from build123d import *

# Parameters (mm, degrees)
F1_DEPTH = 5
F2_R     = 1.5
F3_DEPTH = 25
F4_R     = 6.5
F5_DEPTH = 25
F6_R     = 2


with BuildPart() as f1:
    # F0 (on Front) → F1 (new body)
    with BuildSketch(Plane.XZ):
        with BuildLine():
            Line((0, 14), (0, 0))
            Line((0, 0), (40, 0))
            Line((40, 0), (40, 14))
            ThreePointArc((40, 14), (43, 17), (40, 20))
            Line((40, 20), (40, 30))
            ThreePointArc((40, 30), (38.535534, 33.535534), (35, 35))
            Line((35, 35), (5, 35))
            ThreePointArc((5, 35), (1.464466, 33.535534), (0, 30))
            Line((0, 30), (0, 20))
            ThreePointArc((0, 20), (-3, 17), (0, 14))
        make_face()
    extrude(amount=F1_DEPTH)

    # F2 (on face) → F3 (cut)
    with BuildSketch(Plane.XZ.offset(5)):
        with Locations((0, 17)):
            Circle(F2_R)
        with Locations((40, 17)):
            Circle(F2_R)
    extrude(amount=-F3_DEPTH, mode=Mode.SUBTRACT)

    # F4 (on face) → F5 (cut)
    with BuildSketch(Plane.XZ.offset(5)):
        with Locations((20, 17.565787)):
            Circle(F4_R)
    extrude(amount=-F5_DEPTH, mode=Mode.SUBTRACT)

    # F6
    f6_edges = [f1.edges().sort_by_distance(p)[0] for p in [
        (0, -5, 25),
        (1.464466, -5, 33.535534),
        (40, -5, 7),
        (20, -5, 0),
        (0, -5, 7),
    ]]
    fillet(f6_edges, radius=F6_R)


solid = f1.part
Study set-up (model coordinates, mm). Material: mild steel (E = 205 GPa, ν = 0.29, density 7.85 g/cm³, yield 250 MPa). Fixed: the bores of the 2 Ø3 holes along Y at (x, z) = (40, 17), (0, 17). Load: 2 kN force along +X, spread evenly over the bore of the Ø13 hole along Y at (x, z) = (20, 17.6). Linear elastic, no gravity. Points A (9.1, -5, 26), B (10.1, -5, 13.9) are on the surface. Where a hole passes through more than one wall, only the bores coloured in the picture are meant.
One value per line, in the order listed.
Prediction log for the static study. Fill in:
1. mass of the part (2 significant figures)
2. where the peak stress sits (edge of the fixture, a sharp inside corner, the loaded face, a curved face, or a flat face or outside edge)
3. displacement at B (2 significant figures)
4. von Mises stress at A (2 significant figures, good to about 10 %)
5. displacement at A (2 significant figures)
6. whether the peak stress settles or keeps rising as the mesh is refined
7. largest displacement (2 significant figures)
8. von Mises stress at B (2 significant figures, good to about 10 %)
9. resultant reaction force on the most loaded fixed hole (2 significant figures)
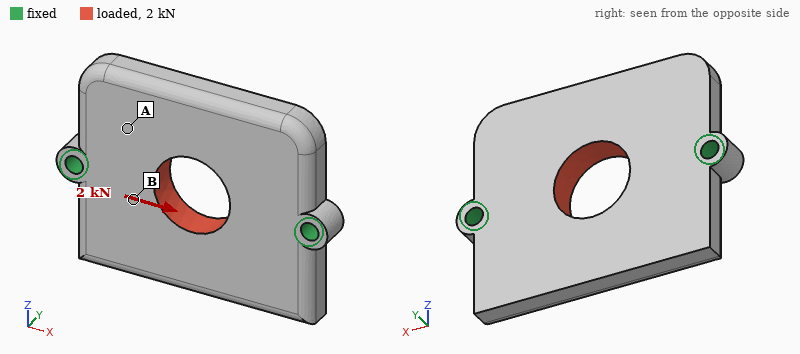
49 g
edge of the fixture
0.96 µm
5.5 MPa
1.2 µm
keeps rising
1.6 µm
14 MPa
1.0 kN
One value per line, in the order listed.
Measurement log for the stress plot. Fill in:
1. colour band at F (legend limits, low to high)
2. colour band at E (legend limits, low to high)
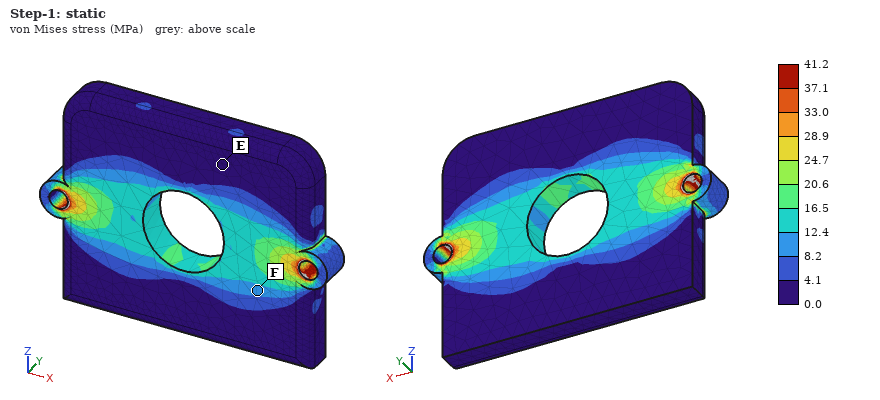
8.2 to 12.4 MPa
0.0 to 4.1 MPa
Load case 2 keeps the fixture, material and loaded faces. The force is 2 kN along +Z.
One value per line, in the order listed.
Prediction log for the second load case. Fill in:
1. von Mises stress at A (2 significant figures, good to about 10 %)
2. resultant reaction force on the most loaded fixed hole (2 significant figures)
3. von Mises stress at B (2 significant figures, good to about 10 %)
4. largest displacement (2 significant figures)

13 MPa
1.0 kN
12 MPa
2.6 µm
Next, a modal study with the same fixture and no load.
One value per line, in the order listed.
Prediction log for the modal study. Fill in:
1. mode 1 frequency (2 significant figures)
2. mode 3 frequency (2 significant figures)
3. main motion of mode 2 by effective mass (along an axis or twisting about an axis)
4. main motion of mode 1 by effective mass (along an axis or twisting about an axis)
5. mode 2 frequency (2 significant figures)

6500 Hz
15 kHz
along Y
twisting about X
8800 Hz
